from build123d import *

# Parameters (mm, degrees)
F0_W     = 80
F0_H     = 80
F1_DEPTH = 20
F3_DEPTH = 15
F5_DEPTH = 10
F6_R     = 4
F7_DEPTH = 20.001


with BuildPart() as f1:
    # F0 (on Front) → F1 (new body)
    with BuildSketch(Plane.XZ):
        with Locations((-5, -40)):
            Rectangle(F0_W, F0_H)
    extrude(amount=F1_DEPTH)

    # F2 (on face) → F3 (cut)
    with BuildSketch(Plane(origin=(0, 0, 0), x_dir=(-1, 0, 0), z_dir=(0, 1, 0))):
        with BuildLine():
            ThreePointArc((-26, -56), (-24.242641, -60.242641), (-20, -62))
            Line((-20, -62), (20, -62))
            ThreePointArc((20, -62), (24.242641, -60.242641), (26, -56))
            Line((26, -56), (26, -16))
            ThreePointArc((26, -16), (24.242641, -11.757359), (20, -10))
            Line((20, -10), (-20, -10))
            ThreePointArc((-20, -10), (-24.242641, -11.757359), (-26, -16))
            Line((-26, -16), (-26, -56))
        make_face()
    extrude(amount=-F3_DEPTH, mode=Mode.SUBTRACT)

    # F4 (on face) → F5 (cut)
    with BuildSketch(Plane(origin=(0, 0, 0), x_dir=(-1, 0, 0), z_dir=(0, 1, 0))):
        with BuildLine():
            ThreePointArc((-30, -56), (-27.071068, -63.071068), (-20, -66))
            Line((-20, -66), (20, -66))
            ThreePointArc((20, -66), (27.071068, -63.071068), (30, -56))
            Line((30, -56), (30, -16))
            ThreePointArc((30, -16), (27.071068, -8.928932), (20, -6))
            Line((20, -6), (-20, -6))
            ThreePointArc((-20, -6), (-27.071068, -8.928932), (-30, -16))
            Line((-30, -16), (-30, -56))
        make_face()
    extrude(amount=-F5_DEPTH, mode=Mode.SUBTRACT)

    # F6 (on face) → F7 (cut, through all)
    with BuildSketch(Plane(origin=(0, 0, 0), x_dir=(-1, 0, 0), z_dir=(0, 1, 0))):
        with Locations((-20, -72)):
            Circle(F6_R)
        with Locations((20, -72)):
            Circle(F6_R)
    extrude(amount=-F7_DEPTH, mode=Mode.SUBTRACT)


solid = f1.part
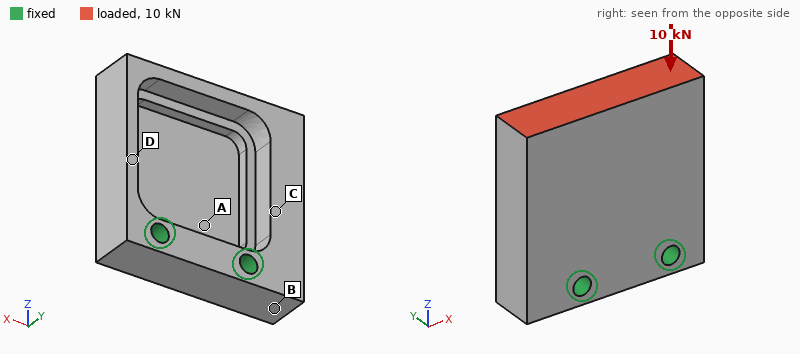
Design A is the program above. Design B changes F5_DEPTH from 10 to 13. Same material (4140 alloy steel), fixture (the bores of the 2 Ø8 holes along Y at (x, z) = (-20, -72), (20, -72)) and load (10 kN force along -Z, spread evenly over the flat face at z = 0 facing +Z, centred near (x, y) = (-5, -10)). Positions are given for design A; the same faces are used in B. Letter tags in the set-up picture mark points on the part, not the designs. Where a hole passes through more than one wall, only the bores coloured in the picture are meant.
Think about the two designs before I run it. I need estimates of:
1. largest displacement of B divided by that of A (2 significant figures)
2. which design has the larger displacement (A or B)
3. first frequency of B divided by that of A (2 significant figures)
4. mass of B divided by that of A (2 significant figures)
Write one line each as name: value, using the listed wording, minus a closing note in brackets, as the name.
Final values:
largest displacement of B divided by that of A: 1.1
which design has the larger displacement: B
first frequency of B divided by that of A: 0.99
mass of B divided by that of A: 0.97
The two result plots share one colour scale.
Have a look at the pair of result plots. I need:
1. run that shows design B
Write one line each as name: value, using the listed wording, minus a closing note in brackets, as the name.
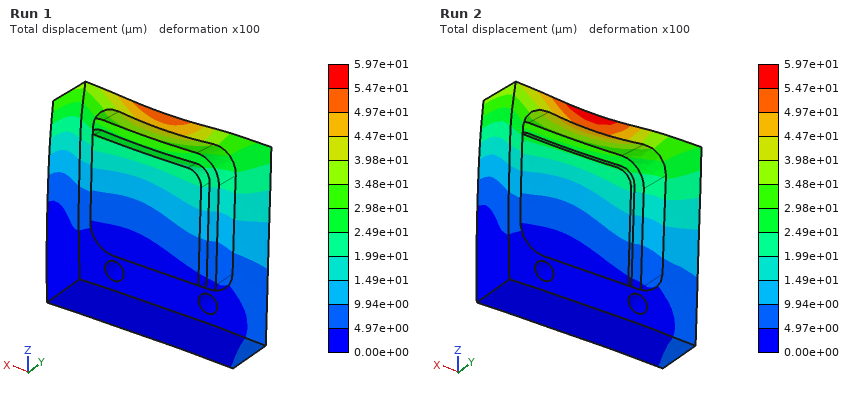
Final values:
run that shows design B: Run 2
